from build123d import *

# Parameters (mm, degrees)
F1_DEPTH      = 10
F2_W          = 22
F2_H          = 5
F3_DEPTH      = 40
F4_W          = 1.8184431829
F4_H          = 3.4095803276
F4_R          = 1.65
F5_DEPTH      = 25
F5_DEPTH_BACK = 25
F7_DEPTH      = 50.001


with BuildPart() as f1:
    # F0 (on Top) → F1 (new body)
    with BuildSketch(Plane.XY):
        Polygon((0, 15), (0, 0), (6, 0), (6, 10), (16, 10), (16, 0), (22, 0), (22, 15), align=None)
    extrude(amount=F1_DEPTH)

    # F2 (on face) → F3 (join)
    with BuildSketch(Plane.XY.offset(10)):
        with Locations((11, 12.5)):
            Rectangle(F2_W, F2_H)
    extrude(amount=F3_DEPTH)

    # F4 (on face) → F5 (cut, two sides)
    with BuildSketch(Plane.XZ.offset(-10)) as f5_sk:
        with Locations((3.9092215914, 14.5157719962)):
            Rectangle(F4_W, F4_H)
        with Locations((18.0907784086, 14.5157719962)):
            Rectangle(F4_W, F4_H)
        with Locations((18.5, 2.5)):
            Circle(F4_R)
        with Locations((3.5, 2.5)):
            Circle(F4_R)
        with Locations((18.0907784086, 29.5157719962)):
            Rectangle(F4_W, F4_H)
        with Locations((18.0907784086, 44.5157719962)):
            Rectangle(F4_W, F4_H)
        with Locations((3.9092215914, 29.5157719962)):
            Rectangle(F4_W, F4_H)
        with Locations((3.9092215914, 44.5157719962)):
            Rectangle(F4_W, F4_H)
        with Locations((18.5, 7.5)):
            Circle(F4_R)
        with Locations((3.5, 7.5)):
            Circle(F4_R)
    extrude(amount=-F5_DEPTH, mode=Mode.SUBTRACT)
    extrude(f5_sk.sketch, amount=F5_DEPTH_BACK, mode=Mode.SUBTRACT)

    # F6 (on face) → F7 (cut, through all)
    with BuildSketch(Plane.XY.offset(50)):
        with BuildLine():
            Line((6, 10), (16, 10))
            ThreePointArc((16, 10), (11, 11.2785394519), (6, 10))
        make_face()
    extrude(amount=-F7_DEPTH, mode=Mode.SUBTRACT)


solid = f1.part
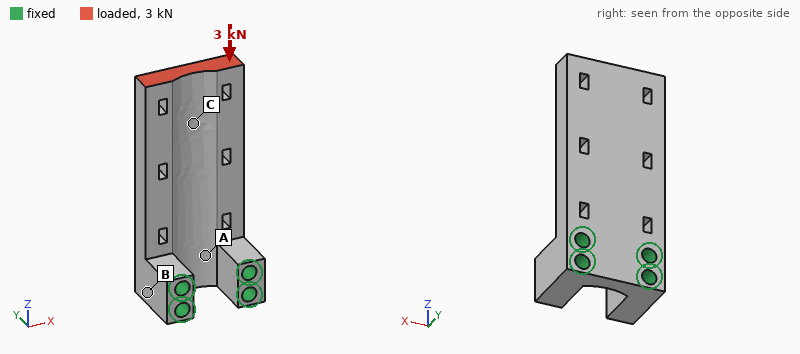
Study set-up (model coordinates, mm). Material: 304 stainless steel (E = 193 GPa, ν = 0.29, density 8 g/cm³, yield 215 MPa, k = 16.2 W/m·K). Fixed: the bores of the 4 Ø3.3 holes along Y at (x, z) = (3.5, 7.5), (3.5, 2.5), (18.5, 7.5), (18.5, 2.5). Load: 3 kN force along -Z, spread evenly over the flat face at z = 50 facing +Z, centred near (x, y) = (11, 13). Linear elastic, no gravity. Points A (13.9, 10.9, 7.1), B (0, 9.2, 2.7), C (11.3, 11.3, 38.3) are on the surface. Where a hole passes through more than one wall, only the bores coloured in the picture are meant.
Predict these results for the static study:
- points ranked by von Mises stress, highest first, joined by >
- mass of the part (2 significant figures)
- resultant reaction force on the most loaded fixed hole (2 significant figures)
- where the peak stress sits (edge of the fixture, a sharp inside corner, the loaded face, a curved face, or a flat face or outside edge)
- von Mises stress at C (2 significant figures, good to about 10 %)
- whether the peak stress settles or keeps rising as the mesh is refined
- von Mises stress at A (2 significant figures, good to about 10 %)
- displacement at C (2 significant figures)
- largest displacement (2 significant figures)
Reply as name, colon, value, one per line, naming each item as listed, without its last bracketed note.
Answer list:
points ranked by von Mises stress, highest first, joined by >: C > A > B
mass of the part: 45 g
resultant reaction force on the most loaded fixed hole: 1.3 kN
where the peak stress sits: edge of the fixture
von Mises stress at C: 33 MPa
whether the peak stress settles or keeps rising as the mesh is refined: keeps rising
von Mises stress at A: 16 MPa
displacement at C: 5.3 µm
largest displacement: 7.5 µm
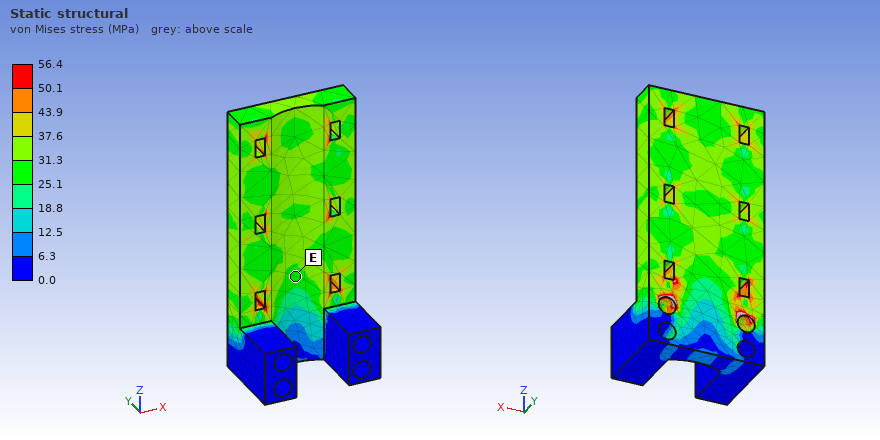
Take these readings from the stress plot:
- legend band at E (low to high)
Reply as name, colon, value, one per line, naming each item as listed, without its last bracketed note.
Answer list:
legend band at E: 25.1 to 31.3 MPa
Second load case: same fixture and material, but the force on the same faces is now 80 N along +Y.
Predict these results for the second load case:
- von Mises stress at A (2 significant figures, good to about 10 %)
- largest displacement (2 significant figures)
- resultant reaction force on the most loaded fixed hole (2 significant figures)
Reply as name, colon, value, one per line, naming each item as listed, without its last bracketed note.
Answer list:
von Mises stress at A: 10 MPa
largest displacement: 58 µm
resultant reaction force on the most loaded fixed hole: 86 N
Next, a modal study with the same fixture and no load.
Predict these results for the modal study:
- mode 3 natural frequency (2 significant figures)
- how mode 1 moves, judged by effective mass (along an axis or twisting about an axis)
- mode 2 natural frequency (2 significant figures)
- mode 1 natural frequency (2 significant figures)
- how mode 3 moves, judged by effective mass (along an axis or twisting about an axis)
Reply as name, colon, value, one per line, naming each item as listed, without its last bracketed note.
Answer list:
mode 3 natural frequency: 8300 Hz
how mode 1 moves, judged by effective mass: along Y
mode 2 natural frequency: 7400 Hz
mode 1 natural frequency: 2100 Hz
how mode 3 moves, judged by effective mass: along X
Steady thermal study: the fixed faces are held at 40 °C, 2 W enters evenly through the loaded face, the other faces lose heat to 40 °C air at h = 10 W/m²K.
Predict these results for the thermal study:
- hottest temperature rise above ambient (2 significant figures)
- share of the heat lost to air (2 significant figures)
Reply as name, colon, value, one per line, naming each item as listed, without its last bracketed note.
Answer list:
hottest temperature rise above ambient: 45 K
share of the heat lost to air: 27 %
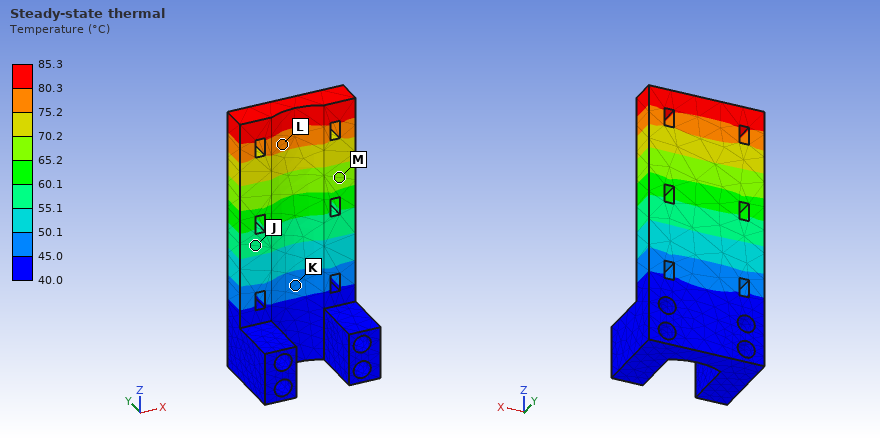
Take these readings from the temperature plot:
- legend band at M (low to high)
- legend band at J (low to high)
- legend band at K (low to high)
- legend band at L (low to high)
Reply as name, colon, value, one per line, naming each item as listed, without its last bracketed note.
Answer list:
legend band at M: 65.2 to 70.2 °C
legend band at J: 55.1 to 60.1 °C
legend band at K: 45.0 to 50.1 °C
legend band at L: 75.2 to 80.3 °C
